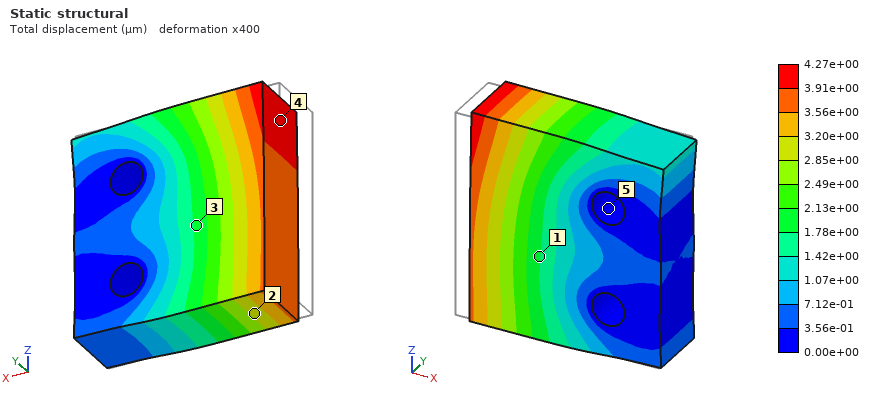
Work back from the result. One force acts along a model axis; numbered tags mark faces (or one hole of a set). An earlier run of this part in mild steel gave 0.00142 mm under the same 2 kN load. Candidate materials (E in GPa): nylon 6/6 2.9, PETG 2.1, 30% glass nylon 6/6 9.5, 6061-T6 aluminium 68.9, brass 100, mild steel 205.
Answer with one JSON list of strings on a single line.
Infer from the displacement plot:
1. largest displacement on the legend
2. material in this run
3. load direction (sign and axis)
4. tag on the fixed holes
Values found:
["4.27e+00 µm", "6061-T6 aluminium", "+X", "5"]
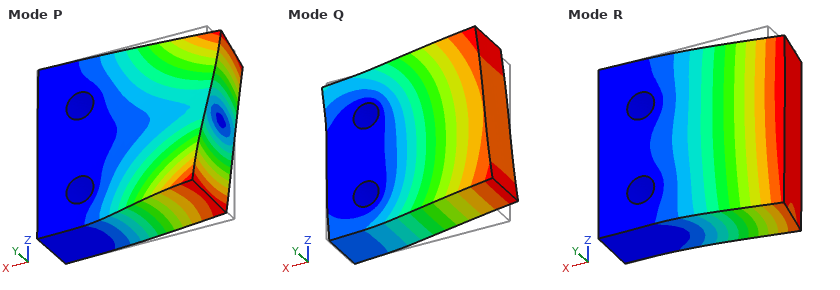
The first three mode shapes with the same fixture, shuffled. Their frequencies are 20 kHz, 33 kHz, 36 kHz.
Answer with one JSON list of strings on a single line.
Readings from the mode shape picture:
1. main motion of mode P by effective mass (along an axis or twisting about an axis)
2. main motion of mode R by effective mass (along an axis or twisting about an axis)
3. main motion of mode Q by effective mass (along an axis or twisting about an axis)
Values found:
["twisting about X", "along Y", "along Z"]
